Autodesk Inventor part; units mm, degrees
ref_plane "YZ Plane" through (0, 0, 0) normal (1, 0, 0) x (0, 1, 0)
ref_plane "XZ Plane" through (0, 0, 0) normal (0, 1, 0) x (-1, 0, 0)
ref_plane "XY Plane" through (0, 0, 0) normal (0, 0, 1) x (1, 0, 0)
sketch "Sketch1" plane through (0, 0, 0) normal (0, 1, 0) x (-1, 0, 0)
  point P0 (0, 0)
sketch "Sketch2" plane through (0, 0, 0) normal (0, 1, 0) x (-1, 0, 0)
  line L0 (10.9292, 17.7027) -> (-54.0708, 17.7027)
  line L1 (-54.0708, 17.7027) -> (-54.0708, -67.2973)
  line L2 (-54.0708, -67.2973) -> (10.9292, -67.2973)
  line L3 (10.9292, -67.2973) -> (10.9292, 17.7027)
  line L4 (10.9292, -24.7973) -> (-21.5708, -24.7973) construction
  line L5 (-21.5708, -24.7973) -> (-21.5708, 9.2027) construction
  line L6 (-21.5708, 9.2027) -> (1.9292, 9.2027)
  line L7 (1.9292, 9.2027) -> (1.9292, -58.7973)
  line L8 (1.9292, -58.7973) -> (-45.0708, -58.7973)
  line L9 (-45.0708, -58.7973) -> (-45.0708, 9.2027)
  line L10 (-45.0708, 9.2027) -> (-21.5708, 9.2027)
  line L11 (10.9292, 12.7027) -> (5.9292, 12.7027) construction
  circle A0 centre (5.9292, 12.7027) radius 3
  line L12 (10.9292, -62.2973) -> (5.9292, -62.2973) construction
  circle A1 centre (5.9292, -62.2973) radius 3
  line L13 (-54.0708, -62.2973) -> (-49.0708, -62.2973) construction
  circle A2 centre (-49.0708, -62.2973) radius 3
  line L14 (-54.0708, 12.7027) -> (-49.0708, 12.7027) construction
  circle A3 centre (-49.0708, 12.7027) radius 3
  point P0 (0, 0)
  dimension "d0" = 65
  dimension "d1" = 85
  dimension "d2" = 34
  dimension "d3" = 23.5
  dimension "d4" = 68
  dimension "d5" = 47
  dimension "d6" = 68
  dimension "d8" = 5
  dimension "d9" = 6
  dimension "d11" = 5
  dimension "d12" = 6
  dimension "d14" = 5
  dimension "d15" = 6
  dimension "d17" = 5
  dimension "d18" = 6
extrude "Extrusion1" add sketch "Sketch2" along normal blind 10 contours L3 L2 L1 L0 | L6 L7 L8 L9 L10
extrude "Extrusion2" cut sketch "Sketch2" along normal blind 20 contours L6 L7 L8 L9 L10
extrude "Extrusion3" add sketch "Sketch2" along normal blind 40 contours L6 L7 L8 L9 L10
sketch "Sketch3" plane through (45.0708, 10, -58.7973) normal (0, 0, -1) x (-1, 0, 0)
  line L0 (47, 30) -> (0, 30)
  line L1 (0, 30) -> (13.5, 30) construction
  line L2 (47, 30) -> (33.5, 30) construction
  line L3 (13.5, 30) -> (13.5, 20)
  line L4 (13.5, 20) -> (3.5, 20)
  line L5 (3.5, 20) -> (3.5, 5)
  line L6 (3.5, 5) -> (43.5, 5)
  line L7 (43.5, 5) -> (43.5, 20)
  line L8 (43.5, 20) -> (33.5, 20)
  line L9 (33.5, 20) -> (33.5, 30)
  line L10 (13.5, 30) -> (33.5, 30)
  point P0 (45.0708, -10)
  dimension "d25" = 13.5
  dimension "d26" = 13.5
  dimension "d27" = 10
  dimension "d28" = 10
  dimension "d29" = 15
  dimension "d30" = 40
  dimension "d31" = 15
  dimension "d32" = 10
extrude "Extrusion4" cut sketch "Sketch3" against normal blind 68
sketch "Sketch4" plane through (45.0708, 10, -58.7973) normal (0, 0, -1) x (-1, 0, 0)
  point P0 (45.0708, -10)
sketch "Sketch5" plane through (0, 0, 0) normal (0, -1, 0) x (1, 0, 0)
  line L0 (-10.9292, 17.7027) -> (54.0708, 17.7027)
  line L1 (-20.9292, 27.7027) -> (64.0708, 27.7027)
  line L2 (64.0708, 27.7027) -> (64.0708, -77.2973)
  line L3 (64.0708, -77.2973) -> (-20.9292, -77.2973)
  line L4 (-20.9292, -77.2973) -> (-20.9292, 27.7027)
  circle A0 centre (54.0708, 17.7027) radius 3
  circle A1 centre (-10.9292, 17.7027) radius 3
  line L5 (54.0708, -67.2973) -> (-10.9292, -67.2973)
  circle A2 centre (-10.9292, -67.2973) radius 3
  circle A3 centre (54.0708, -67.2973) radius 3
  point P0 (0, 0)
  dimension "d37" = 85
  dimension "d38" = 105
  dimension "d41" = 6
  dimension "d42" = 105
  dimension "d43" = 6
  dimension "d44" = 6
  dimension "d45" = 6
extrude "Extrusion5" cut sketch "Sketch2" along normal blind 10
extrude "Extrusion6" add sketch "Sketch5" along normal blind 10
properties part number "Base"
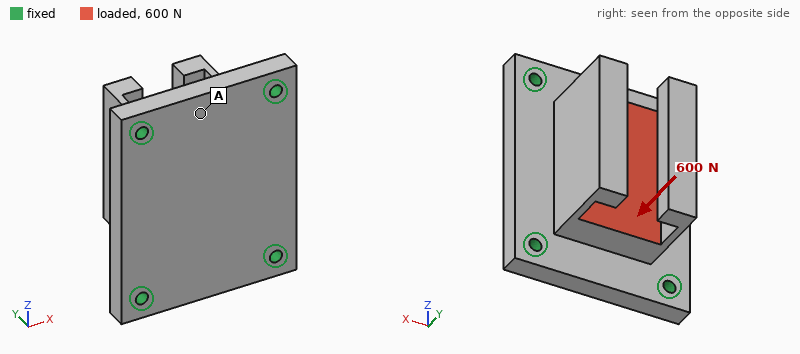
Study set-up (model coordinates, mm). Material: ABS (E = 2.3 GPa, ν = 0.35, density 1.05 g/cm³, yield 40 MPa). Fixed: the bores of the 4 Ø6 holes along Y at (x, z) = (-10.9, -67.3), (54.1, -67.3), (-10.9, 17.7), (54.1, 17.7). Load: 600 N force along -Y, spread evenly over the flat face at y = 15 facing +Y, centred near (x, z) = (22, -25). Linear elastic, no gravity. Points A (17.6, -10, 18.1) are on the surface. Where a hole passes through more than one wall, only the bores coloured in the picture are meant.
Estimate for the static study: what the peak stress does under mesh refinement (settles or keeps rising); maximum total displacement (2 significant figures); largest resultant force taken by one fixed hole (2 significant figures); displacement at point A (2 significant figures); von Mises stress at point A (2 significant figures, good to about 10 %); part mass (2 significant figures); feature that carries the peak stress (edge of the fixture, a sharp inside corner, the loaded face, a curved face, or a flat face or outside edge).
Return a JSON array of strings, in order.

["keeps rising", "48 µm", "160 N", "30 µm", "0.82 MPa", "170 g", "edge of the fixture"]
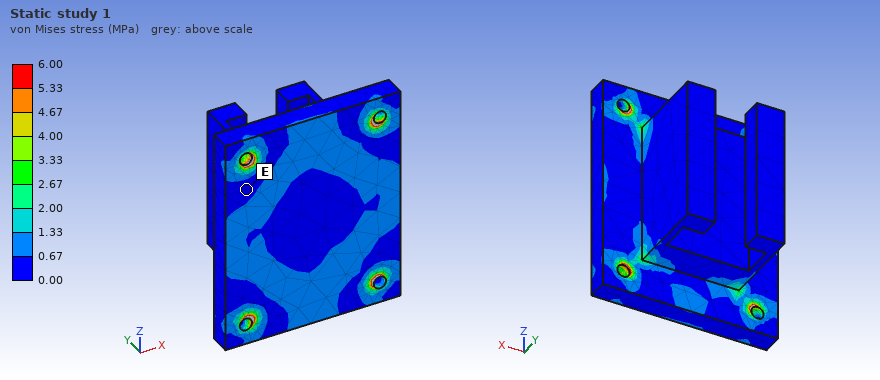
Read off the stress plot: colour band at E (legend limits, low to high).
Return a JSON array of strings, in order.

["0.00 to 0.67 MPa"]
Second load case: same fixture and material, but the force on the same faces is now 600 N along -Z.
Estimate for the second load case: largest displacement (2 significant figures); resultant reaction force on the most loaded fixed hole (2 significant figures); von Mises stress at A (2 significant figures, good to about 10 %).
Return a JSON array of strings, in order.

["35 µm", "180 N", "0.57 MPa"]
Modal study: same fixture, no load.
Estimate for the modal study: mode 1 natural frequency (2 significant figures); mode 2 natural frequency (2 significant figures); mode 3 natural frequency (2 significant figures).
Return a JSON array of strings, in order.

["620 Hz", "630 Hz", "1400 Hz"]
